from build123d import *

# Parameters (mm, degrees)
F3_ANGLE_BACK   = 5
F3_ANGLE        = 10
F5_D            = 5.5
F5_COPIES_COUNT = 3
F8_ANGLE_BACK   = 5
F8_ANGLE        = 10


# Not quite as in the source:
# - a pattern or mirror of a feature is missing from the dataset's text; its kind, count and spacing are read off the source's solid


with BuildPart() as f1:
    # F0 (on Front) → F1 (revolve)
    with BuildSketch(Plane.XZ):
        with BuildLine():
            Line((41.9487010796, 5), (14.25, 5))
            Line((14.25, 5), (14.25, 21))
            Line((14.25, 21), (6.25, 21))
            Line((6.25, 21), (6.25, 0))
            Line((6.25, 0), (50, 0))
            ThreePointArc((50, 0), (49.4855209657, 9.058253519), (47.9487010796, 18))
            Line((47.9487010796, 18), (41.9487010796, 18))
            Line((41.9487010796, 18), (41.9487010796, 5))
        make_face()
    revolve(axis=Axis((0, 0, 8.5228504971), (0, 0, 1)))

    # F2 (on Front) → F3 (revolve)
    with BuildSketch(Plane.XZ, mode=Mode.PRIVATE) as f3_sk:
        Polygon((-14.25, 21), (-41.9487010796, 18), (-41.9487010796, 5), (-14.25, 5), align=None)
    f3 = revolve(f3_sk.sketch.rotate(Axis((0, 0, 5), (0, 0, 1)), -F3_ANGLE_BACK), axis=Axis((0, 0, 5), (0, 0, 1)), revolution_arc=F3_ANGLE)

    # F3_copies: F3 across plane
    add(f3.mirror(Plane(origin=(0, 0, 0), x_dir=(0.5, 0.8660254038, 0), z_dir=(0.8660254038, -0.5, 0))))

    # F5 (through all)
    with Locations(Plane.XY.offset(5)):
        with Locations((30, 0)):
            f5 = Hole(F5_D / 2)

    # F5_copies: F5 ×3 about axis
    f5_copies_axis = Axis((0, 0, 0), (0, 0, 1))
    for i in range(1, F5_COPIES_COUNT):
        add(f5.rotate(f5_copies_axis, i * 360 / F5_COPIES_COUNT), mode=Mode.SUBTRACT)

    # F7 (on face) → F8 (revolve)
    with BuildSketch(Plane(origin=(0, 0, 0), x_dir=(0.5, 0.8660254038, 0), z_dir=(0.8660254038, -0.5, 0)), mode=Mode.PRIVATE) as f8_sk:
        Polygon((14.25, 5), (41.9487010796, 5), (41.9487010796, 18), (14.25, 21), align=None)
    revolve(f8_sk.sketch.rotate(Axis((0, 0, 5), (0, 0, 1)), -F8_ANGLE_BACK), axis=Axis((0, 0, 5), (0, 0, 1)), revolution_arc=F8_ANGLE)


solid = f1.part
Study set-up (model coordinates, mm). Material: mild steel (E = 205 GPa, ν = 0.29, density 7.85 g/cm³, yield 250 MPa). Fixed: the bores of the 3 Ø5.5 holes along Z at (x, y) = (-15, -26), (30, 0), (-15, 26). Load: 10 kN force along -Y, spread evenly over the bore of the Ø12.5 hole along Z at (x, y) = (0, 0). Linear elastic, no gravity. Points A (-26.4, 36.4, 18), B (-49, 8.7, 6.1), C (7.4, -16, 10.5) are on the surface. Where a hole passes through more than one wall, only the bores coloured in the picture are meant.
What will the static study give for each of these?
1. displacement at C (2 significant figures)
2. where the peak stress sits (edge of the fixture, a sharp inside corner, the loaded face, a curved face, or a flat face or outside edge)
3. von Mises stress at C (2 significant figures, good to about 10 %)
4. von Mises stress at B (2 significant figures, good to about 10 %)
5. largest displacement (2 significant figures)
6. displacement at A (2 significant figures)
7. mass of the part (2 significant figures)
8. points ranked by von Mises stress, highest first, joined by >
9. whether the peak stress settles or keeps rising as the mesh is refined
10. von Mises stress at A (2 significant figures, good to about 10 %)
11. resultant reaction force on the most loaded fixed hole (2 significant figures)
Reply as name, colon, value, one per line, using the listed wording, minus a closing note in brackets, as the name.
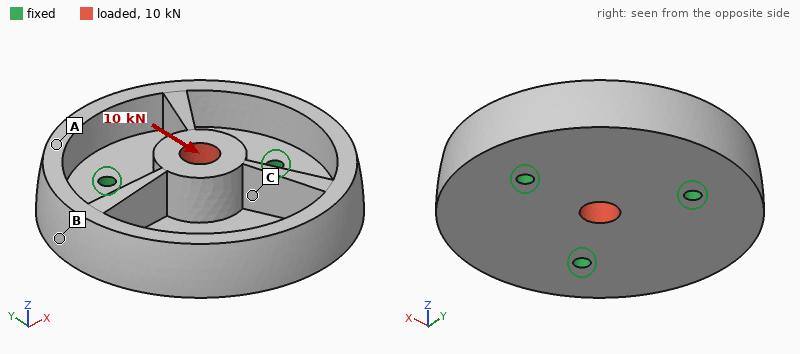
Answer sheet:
displacement at C: 10 µm
where the peak stress sits: edge of the fixture
von Mises stress at C: 31 MPa
von Mises stress at B: 8.2 MPa
largest displacement: 18 µm
displacement at A: 3.8 µm
mass of the part: 620 g
points ranked by von Mises stress, highest first, joined by >: C > A > B
whether the peak stress settles or keeps rising as the mesh is refined: keeps rising
von Mises stress at A: 16 MPa
resultant reaction force on the most loaded fixed hole: 3.6 kN
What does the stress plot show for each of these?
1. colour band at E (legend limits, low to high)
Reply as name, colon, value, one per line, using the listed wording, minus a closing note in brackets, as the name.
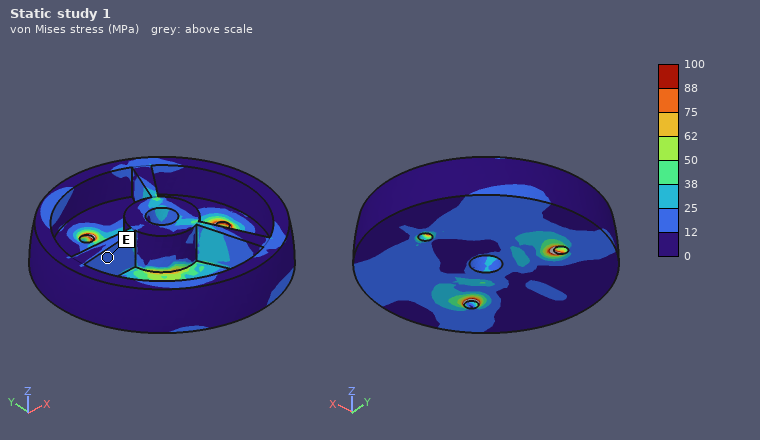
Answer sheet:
colour band at E: 12 to 25 MPa
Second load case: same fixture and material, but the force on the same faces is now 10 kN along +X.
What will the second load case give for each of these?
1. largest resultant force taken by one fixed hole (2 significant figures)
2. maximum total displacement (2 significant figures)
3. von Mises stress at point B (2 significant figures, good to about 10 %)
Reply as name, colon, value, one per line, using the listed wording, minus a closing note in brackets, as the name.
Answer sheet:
largest resultant force taken by one fixed hole: 3.8 kN
maximum total displacement: 20 µm
von Mises stress at point B: 11 MPa
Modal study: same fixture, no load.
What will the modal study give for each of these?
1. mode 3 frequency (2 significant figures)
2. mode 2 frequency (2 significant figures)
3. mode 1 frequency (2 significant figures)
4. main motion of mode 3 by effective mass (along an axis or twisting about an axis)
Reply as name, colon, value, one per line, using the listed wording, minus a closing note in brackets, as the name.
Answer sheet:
mode 3 frequency: 5900 Hz
mode 2 frequency: 4100 Hz
mode 1 frequency: 4100 Hz
main motion of mode 3 by effective mass: along Z
